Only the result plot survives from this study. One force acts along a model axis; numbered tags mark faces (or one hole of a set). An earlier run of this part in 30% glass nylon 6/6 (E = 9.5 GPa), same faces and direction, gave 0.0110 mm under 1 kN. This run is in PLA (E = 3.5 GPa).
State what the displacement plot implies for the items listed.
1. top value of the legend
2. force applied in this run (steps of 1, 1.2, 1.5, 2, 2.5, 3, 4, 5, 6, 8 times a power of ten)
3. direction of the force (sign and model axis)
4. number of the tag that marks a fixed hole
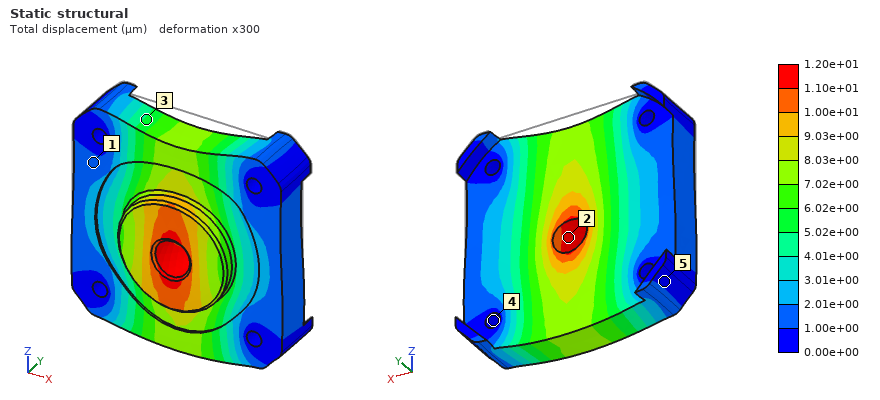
1.20e+01 µm
400 N
-Z
4
